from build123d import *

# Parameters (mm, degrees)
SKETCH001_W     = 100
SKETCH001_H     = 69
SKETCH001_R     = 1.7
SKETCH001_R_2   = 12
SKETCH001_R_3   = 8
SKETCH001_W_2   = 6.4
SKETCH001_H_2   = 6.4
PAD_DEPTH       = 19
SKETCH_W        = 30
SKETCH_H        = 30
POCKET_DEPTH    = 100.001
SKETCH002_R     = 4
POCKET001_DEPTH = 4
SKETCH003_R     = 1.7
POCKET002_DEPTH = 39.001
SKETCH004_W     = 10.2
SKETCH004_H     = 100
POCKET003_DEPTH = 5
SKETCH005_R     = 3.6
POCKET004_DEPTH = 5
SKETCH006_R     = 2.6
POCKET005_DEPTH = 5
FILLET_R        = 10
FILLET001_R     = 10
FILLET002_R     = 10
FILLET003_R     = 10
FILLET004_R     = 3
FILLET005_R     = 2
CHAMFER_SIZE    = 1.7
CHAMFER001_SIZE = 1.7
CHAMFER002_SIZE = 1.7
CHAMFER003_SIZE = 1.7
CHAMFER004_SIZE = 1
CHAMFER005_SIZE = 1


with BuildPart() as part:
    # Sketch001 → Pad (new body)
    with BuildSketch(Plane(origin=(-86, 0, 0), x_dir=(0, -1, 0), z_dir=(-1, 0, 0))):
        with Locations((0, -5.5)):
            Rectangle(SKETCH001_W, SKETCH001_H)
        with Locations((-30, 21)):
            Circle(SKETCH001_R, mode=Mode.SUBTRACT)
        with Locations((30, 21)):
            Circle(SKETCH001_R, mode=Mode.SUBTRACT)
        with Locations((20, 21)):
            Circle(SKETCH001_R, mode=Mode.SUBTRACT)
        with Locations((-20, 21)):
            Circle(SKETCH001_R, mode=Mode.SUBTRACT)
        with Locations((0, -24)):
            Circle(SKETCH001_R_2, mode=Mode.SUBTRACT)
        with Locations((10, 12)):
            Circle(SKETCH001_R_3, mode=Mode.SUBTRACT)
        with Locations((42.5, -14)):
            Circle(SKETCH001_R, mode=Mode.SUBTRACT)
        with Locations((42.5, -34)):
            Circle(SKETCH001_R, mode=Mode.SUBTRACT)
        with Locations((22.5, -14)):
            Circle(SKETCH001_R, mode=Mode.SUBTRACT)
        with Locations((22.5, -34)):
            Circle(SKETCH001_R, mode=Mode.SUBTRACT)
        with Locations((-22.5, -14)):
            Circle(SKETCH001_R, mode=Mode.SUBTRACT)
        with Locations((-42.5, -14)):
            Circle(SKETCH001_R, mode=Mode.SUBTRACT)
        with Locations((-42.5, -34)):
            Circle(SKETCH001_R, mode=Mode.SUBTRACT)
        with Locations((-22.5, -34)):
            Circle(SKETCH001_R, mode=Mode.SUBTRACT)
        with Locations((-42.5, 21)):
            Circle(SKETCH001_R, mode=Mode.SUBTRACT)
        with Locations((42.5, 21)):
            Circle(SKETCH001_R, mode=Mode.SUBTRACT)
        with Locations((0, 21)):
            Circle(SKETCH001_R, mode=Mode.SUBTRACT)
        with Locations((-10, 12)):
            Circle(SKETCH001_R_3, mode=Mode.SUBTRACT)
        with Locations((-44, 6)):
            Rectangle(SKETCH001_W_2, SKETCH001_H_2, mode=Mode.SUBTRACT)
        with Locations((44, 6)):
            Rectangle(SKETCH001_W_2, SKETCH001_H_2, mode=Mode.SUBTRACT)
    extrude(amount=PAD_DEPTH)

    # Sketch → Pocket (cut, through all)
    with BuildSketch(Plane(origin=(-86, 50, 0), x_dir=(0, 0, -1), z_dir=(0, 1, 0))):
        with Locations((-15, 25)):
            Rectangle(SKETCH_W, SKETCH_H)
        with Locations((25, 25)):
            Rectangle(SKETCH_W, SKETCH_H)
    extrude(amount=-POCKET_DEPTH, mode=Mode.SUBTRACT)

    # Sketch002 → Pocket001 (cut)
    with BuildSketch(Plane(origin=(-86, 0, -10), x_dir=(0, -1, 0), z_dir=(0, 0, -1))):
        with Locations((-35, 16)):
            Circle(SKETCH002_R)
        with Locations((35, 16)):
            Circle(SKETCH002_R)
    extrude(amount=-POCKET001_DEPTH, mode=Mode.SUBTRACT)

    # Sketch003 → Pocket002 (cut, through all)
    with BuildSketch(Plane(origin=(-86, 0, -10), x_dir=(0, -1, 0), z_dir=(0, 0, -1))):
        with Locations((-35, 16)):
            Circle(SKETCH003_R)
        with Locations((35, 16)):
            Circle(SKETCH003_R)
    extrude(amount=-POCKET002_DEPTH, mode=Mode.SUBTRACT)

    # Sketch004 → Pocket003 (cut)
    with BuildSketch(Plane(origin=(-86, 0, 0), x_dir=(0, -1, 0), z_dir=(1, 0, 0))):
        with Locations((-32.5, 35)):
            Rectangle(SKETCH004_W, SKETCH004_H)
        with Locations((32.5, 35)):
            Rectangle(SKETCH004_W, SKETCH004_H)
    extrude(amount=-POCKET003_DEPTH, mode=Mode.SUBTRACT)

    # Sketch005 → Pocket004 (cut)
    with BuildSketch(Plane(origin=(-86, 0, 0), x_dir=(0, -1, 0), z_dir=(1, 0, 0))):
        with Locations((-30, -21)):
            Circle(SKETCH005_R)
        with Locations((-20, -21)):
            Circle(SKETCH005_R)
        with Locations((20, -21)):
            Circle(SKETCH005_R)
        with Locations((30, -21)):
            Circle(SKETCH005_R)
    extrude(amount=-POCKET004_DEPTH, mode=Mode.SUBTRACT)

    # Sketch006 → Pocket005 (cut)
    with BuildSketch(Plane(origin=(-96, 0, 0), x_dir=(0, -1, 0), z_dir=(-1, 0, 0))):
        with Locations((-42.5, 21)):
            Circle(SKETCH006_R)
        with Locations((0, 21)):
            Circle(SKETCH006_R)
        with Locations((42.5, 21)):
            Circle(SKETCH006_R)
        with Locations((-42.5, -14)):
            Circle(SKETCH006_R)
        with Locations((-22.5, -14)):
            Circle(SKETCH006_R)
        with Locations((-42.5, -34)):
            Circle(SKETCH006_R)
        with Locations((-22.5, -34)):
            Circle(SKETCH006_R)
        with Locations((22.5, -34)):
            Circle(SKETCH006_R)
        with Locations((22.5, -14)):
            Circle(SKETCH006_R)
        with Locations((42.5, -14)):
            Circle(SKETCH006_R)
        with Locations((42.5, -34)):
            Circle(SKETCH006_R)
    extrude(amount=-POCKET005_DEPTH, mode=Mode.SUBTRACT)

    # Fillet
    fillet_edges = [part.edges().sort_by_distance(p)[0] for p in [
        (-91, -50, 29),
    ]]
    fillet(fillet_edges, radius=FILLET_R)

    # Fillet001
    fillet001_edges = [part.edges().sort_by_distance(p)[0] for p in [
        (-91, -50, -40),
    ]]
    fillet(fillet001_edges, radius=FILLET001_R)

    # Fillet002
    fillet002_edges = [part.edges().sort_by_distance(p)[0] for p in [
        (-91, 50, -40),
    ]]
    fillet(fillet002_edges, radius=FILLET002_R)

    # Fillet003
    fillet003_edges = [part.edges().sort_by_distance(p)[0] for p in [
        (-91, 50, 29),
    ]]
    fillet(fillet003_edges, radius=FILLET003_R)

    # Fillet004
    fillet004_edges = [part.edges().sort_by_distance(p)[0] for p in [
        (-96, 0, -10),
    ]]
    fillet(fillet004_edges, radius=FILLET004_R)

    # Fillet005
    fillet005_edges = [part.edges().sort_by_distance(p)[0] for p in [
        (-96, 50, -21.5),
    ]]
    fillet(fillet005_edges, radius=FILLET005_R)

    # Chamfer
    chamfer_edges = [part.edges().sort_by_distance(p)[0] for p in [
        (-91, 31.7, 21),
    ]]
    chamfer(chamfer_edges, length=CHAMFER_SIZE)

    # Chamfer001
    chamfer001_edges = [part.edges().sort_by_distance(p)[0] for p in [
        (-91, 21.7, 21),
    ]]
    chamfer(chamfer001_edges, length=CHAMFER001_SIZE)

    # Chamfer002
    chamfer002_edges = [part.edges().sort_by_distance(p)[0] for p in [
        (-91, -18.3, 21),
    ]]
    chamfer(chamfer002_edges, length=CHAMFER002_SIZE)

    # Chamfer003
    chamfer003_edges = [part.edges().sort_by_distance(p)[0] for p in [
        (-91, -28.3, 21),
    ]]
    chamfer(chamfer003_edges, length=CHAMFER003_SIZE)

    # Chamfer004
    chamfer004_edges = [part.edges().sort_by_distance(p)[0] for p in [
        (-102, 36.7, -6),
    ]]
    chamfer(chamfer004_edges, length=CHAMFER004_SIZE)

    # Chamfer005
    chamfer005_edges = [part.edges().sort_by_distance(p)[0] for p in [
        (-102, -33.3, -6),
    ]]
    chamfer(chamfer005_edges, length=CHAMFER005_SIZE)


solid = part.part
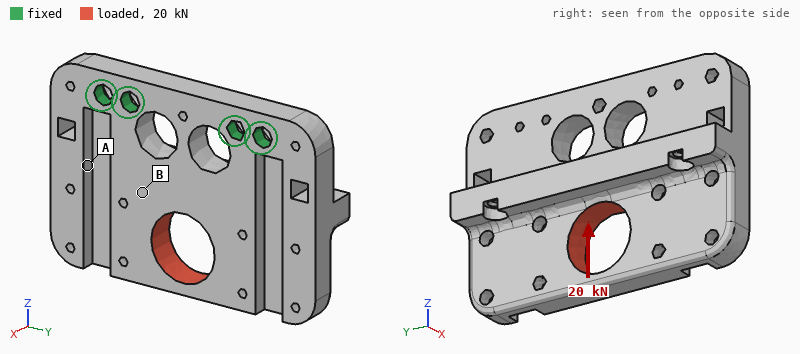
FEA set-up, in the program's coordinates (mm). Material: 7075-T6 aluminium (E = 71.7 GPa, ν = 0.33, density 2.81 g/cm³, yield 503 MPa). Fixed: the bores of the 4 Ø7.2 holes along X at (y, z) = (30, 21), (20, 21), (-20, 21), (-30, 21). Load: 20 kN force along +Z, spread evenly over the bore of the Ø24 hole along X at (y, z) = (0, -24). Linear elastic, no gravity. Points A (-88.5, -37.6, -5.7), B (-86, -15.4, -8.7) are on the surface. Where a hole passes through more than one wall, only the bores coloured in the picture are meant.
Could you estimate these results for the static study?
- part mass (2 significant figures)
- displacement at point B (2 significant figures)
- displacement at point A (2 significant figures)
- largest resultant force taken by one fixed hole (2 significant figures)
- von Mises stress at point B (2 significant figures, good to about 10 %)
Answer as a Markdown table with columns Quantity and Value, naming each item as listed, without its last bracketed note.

| Quantity | Value |
|---|---|
| part mass | 170 g |
| displacement at point B | 27 µm |
| displacement at point A | 18 µm |
| largest resultant force taken by one fixed hole | 5.3 kN |
| von Mises stress at point B | 56 MPa |
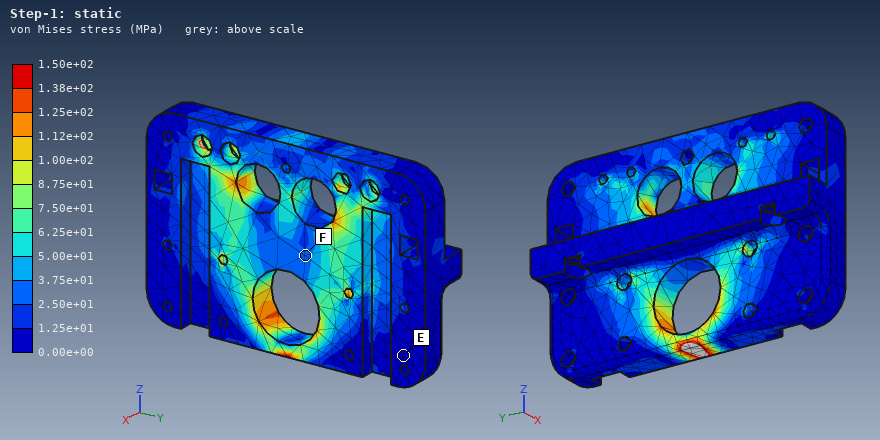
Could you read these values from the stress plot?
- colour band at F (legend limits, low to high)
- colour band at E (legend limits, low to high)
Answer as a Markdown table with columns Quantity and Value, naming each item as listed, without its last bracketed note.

| Quantity | Value |
|---|---|
| colour band at F | 2.50e+01 to 3.75e+01 MPa |
| colour band at E | 0.00e+00 to 1.25e+01 MPa |
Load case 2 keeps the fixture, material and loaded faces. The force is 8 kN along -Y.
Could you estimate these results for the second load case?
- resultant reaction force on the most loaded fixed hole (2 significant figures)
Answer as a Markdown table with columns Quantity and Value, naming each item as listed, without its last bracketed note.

| Quantity | Value |
|---|---|
| resultant reaction force on the most loaded fixed hole | 6.0 kN |
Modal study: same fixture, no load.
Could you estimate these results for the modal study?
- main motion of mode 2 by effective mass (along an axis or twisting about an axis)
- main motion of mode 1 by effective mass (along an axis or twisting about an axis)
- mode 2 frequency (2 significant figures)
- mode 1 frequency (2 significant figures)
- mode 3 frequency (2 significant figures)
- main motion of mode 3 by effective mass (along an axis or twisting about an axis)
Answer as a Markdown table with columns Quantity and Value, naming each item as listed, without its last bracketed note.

| Quantity | Value |
|---|---|
| main motion of mode 2 by effective mass | twisting about Z |
| main motion of mode 1 by effective mass | along X |
| mode 2 frequency | 3000 Hz |
| mode 1 frequency | 1700 Hz |
| mode 3 frequency | 6100 Hz |
| main motion of mode 3 by effective mass | along Y |
